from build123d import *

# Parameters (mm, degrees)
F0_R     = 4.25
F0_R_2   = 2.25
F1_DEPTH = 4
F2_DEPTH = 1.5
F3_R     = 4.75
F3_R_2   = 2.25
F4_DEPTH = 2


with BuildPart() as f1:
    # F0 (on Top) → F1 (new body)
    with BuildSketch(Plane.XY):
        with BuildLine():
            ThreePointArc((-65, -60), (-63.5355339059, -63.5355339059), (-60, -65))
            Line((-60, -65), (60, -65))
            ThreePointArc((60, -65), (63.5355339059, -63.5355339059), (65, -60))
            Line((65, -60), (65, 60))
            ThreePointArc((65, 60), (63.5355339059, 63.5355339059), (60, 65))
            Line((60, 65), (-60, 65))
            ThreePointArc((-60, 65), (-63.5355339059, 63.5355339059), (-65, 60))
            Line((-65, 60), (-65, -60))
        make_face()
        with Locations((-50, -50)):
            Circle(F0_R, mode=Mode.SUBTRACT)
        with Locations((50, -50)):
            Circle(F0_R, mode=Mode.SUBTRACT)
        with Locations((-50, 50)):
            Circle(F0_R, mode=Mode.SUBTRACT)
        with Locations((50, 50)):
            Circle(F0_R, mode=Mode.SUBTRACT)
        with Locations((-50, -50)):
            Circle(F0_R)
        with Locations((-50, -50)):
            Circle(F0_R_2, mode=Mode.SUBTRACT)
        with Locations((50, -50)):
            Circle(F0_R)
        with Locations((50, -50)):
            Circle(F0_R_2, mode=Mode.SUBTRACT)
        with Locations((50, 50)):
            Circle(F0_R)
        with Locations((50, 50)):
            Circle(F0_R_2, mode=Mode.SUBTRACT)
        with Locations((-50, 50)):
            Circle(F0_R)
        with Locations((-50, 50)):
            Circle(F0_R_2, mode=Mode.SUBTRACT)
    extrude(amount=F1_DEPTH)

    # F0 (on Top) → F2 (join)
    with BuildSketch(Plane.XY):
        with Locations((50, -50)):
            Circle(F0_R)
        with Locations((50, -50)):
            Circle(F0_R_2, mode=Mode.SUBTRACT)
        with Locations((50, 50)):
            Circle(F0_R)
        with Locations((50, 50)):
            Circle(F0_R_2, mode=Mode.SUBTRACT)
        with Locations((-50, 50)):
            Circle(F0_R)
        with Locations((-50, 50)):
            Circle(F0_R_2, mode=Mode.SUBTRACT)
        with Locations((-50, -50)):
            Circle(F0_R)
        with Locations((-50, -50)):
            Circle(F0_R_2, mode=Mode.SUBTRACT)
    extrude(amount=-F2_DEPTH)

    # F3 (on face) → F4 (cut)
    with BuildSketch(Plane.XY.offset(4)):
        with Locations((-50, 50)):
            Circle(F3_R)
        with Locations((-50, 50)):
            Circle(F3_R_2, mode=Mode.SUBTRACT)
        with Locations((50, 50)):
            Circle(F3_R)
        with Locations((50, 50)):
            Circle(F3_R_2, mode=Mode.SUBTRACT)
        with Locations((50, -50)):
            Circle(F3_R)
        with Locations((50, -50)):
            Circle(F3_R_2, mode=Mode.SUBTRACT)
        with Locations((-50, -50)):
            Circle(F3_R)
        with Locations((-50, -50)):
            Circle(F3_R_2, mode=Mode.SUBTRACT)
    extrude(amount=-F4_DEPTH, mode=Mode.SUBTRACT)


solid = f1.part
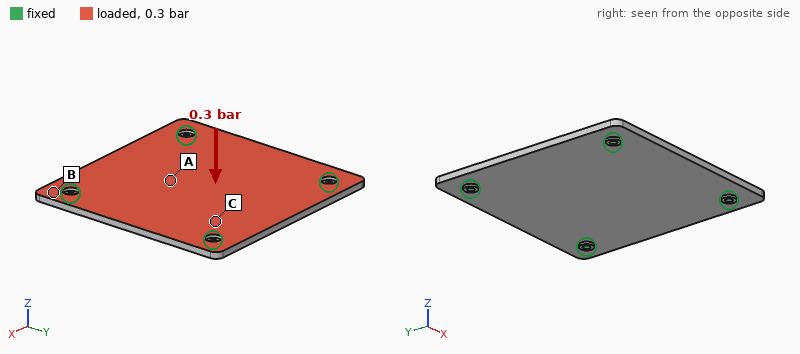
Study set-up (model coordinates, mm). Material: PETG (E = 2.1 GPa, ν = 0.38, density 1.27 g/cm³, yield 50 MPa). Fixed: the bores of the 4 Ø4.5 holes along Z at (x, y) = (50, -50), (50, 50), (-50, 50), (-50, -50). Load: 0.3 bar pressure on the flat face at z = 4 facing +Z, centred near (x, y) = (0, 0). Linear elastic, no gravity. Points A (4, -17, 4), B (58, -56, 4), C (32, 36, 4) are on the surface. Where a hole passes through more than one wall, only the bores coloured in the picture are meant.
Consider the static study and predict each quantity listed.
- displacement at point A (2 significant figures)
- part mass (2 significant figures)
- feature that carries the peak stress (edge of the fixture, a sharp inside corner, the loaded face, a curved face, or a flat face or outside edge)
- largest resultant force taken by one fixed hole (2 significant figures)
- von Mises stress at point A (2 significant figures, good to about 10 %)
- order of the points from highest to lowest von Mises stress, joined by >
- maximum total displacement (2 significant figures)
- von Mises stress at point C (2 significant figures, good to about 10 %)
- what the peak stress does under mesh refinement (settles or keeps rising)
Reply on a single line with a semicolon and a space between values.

1.9 mm; 85 g; edge of the fixture; 240 N; 6.7 MPa; A > C > B; 2.0 mm; 3.7 MPa; keeps rising
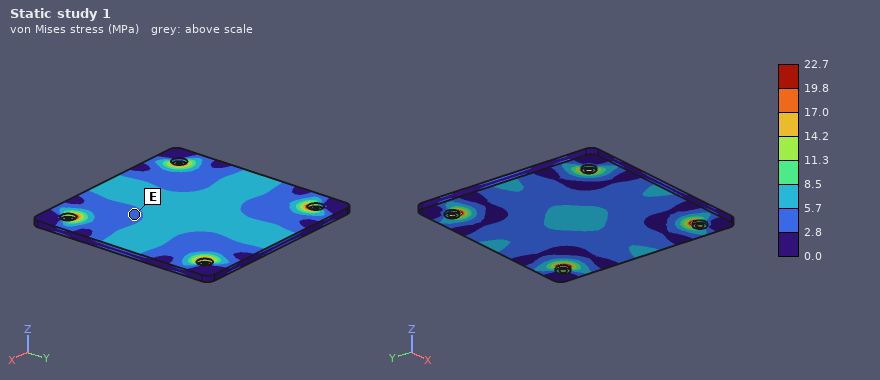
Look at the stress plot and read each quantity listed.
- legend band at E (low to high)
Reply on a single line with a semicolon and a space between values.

2.8 to 5.7 MPa
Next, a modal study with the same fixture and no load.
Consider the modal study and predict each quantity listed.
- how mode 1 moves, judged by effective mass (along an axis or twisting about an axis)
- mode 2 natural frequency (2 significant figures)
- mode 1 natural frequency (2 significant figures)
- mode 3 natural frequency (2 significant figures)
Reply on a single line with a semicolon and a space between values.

along Z; 520 Hz; 330 Hz; 520 Hz
